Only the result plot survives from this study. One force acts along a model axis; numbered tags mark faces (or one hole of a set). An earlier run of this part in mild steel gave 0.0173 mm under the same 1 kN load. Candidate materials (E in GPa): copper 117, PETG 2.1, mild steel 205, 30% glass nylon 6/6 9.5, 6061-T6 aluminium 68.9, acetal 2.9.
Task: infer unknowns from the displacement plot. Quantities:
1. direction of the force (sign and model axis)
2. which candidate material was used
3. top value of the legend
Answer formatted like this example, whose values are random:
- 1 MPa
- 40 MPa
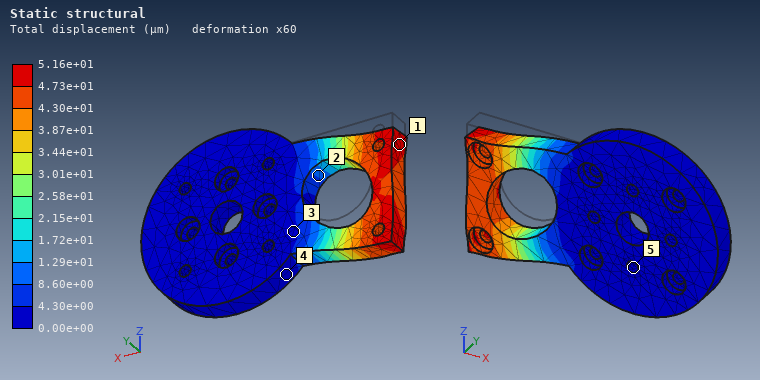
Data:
- -Z
- 6061-T6 aluminium
- 5.16e+01 µm
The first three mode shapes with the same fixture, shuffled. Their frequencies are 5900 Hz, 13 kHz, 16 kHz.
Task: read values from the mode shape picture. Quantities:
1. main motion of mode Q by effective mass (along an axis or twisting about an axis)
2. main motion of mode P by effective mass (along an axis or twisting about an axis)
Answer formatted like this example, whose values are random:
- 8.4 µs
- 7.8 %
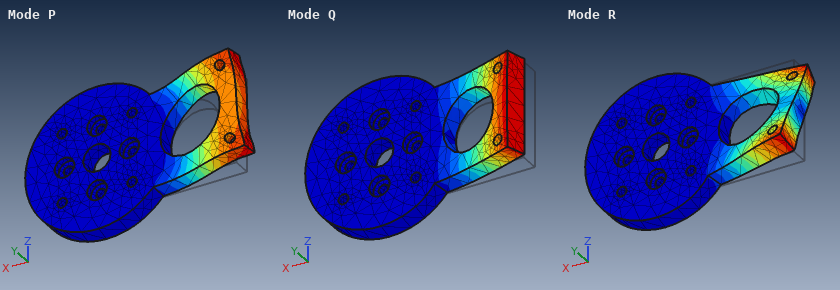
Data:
- along Y
- along Z
